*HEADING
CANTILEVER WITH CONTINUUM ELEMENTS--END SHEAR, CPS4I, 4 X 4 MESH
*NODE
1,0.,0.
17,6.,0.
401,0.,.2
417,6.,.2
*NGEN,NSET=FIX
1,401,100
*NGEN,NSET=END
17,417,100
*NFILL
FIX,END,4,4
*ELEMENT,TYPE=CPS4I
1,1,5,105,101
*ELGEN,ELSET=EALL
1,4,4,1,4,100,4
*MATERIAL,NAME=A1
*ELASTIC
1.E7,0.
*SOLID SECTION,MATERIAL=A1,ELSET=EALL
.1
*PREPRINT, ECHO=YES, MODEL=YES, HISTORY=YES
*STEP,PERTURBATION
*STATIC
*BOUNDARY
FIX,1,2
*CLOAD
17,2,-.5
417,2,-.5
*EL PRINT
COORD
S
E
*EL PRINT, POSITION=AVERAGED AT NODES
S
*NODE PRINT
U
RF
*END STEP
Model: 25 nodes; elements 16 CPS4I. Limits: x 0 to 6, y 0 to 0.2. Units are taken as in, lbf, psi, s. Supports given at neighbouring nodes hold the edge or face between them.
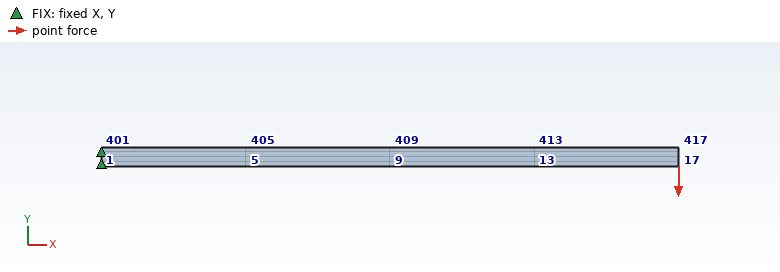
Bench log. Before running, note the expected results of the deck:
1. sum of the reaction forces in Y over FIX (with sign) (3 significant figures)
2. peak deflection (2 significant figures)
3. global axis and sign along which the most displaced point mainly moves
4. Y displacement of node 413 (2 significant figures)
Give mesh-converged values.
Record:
1.00 lbf
0.11 in
-Y
-0.068 in
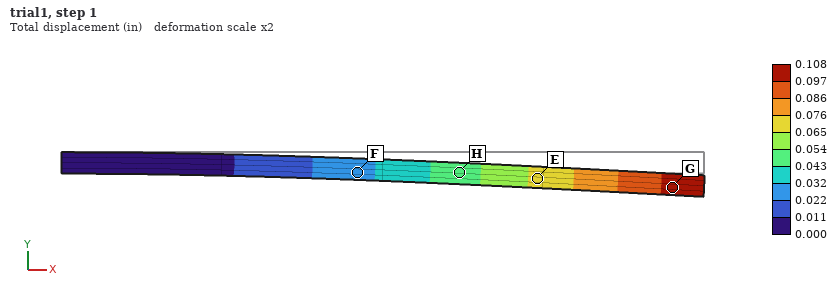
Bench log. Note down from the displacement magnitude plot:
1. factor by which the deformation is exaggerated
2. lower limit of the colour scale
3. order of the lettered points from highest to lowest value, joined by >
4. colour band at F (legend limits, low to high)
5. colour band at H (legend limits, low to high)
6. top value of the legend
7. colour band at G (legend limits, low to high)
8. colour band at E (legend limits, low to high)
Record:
2
0.000 in
G > E > H > F
0.022 to 0.032 in
0.043 to 0.054 in
0.108 in
0.097 to 0.108 in
0.065 to 0.076 in
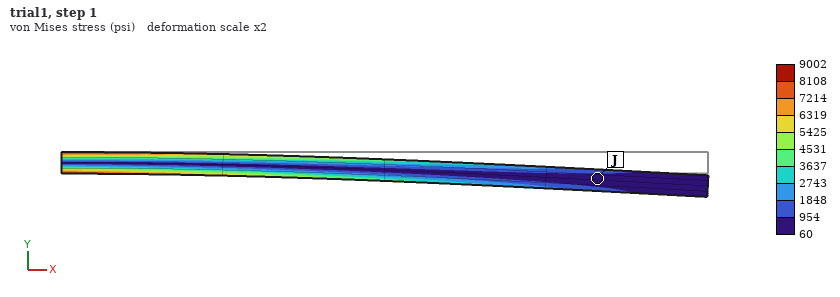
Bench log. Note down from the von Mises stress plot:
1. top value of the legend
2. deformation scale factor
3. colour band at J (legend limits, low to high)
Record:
9002 psi
2
60 to 954 psi
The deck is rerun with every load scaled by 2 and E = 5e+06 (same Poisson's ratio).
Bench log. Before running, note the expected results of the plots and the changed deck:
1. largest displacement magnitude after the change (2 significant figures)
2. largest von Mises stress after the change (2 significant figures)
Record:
0.43 in
18000 psi
